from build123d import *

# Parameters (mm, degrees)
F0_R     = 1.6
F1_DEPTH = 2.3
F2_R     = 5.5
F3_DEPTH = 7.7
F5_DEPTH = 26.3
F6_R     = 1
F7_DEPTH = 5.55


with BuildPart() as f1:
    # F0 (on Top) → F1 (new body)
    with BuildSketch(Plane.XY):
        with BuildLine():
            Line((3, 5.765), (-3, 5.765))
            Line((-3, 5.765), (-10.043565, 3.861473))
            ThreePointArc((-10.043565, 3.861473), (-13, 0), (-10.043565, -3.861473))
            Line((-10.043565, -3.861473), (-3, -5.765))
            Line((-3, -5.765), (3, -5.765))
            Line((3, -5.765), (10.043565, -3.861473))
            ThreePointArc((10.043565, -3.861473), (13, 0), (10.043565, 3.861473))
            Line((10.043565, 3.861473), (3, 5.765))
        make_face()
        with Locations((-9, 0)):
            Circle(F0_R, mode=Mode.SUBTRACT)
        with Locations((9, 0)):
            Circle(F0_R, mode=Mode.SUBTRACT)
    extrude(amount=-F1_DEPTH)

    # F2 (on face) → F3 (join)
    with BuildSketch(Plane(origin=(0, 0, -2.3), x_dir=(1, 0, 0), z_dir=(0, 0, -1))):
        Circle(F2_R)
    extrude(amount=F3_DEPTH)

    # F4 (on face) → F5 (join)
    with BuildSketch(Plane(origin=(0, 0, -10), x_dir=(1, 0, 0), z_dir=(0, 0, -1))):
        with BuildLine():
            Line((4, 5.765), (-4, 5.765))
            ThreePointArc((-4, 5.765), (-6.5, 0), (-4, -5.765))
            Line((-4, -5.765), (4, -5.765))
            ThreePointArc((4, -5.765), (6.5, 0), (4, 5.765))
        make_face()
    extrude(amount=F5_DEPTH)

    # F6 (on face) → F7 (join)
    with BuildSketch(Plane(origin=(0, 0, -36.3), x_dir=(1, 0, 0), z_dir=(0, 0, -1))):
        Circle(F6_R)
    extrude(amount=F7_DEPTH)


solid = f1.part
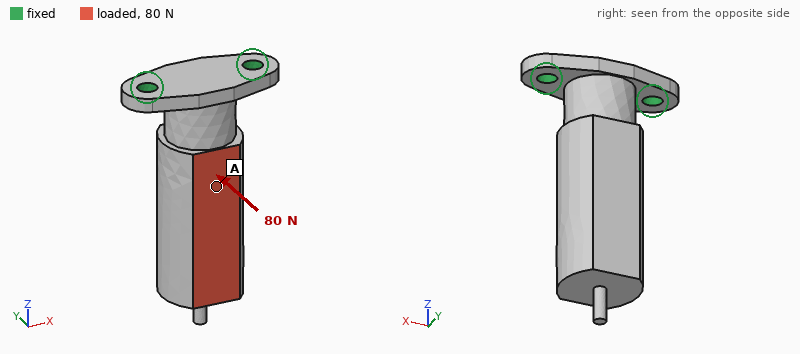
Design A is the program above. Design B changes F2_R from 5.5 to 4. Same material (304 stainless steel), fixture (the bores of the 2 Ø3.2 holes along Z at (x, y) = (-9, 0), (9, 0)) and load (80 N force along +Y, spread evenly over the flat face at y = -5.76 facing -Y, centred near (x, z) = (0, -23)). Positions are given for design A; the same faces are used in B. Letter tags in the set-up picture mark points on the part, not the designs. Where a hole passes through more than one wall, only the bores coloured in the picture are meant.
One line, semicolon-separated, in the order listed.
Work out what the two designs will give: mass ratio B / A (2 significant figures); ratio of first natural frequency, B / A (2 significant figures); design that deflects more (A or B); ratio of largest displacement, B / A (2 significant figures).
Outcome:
0.93; 0.79; B; 1.6
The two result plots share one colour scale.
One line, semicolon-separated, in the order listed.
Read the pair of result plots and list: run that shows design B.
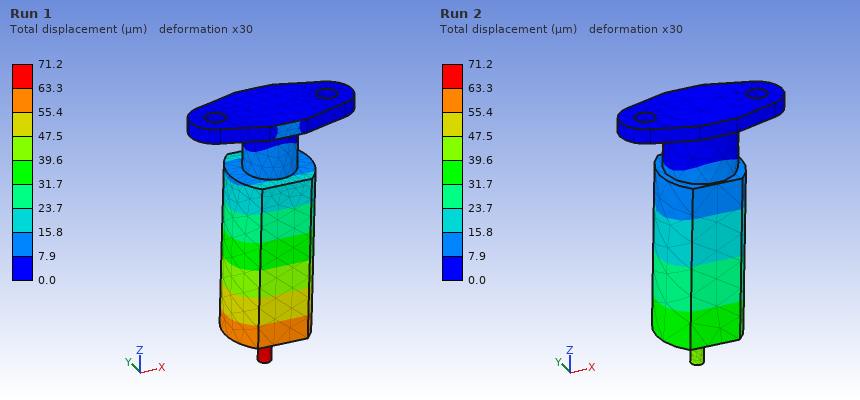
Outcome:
Run 1
